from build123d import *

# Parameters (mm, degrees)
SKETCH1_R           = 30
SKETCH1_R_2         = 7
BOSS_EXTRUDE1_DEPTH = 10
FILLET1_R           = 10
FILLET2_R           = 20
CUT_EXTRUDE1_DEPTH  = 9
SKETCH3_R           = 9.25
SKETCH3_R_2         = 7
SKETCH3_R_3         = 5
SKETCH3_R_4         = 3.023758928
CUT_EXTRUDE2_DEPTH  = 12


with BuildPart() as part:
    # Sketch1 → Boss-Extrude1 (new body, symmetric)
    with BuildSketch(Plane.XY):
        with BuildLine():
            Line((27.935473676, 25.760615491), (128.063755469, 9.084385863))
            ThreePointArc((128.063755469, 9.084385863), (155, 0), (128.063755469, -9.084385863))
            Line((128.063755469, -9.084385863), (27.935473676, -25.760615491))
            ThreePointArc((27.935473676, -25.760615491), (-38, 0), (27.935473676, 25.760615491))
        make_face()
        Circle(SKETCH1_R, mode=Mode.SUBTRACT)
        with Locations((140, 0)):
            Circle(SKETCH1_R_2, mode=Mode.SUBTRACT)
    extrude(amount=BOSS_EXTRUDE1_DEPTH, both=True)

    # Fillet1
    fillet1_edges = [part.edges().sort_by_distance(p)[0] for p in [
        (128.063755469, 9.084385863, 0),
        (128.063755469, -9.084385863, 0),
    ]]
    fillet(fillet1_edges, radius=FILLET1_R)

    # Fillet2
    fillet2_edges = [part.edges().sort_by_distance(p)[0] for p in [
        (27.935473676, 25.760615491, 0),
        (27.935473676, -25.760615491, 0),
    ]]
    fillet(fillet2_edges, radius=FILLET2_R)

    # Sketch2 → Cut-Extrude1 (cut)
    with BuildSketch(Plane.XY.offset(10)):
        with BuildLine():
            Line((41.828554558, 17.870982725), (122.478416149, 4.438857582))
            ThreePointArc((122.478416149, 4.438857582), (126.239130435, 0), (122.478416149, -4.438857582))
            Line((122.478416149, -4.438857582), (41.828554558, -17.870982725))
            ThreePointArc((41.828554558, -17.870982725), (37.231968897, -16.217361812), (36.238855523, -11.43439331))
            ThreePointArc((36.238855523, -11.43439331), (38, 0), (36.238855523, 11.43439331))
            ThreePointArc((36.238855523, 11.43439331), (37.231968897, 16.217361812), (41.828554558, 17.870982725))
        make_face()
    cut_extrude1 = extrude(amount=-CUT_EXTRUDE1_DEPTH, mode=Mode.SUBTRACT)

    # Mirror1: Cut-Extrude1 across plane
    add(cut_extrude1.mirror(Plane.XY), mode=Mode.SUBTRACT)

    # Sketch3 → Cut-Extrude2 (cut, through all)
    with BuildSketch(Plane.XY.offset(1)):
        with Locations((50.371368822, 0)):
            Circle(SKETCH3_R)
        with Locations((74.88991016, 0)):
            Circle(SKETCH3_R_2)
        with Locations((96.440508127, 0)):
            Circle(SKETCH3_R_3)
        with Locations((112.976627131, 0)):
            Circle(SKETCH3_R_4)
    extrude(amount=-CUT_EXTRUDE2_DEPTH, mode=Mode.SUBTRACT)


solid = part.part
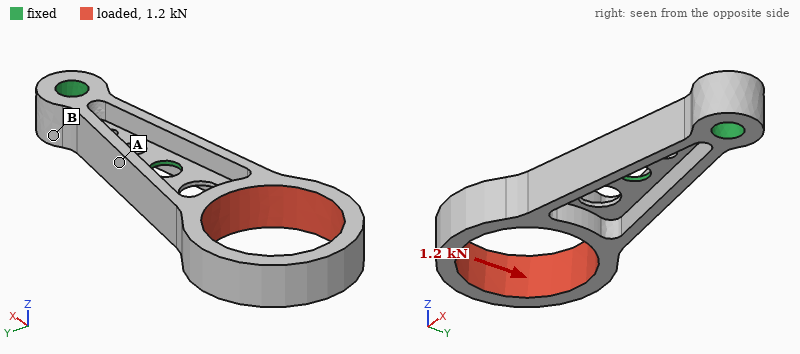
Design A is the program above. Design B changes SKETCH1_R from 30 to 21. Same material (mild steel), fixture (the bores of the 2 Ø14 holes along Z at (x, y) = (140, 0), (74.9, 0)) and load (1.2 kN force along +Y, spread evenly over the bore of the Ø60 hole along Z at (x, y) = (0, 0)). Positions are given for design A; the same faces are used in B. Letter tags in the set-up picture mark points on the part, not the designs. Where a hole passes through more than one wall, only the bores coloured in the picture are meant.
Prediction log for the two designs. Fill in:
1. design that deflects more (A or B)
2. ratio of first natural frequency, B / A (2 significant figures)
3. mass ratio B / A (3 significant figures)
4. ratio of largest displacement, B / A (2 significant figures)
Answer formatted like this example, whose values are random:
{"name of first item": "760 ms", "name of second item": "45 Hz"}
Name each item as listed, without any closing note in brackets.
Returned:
{"design that deflects more": "A", "ratio of first natural frequency, B / A": "0.77", "mass ratio B / A": "1.41", "ratio of largest displacement, B / A": "0.61"}
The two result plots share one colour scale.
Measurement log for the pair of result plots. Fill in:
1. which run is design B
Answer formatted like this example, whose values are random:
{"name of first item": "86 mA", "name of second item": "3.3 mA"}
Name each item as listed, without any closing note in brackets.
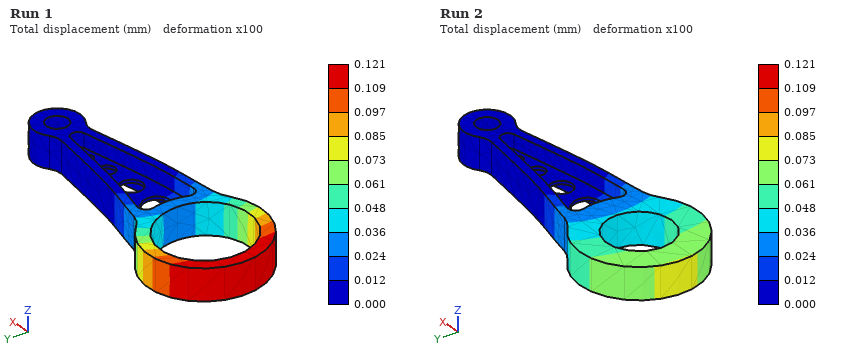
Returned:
{"which run is design B": "Run 2"}
